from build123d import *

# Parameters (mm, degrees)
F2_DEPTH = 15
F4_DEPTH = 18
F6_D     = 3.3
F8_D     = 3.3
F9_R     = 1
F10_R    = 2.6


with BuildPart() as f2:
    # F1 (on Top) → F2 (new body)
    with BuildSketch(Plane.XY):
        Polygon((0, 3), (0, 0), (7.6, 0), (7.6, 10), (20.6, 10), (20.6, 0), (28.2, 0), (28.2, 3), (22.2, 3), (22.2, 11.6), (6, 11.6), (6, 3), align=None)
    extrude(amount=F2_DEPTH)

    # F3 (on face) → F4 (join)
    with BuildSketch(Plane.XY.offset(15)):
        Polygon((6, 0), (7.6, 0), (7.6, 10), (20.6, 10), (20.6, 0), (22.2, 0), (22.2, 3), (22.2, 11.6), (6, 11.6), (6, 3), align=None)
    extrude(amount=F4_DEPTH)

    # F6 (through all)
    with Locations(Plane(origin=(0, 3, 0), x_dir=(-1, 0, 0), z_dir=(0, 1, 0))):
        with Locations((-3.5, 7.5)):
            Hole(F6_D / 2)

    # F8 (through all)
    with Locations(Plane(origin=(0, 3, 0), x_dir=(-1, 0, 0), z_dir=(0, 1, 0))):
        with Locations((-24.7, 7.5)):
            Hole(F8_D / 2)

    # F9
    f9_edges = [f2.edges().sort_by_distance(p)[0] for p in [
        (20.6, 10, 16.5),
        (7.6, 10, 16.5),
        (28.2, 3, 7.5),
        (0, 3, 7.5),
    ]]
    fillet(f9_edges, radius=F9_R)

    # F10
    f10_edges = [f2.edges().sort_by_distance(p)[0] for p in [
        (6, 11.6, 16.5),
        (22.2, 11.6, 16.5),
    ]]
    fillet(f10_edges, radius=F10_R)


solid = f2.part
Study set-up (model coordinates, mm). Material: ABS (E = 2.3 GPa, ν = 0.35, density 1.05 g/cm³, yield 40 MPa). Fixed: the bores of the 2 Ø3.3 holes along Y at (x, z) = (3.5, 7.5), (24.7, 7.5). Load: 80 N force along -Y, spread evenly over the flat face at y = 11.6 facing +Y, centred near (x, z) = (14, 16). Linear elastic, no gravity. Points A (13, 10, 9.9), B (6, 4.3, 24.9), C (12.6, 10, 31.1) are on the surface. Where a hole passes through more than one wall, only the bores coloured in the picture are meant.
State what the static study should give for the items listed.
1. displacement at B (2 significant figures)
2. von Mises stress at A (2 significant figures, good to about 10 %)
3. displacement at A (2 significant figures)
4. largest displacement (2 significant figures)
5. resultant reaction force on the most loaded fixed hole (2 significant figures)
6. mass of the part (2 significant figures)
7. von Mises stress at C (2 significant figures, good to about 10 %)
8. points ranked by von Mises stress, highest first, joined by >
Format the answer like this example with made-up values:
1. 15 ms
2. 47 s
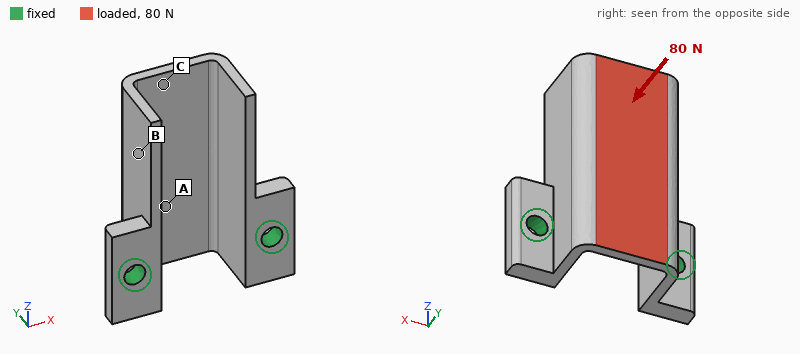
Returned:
1. 0.24 mm
2. 4.6 MPa
3. 0.13 mm
4. 0.49 mm
5. 43 N
6. 2.4 g
7. 7.4 MPa
8. C > A > B
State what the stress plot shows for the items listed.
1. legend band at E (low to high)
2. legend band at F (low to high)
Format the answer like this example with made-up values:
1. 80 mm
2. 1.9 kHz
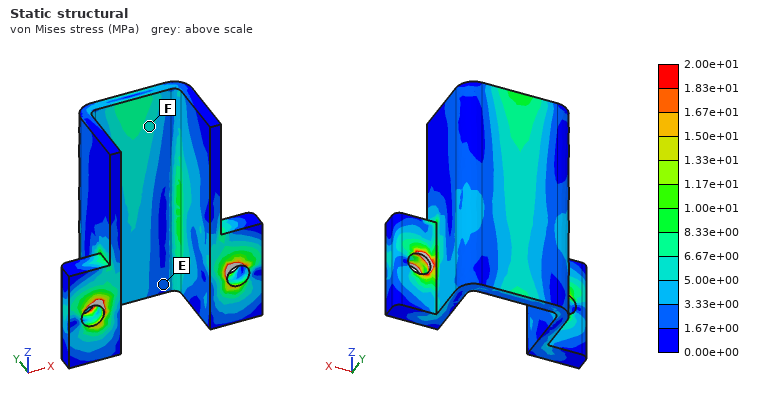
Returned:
1. 1.67e+00 to 3.33e+00 MPa
2. 5.00e+00 to 6.67e+00 MPa
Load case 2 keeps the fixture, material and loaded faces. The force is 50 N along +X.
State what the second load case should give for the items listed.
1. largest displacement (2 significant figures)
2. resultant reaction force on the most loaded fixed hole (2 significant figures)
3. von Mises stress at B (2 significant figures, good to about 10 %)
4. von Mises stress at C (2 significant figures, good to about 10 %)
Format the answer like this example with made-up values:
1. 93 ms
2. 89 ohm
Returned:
1. 0.25 mm
2. 37 N
3. 2.5 MPa
4. 1.5 MPa
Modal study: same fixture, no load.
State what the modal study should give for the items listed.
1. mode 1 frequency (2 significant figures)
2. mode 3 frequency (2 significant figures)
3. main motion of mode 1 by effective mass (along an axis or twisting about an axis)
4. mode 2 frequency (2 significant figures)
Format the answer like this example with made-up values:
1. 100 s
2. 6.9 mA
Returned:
1. 1600 Hz
2. 2900 Hz
3. along X
4. 1800 Hz
